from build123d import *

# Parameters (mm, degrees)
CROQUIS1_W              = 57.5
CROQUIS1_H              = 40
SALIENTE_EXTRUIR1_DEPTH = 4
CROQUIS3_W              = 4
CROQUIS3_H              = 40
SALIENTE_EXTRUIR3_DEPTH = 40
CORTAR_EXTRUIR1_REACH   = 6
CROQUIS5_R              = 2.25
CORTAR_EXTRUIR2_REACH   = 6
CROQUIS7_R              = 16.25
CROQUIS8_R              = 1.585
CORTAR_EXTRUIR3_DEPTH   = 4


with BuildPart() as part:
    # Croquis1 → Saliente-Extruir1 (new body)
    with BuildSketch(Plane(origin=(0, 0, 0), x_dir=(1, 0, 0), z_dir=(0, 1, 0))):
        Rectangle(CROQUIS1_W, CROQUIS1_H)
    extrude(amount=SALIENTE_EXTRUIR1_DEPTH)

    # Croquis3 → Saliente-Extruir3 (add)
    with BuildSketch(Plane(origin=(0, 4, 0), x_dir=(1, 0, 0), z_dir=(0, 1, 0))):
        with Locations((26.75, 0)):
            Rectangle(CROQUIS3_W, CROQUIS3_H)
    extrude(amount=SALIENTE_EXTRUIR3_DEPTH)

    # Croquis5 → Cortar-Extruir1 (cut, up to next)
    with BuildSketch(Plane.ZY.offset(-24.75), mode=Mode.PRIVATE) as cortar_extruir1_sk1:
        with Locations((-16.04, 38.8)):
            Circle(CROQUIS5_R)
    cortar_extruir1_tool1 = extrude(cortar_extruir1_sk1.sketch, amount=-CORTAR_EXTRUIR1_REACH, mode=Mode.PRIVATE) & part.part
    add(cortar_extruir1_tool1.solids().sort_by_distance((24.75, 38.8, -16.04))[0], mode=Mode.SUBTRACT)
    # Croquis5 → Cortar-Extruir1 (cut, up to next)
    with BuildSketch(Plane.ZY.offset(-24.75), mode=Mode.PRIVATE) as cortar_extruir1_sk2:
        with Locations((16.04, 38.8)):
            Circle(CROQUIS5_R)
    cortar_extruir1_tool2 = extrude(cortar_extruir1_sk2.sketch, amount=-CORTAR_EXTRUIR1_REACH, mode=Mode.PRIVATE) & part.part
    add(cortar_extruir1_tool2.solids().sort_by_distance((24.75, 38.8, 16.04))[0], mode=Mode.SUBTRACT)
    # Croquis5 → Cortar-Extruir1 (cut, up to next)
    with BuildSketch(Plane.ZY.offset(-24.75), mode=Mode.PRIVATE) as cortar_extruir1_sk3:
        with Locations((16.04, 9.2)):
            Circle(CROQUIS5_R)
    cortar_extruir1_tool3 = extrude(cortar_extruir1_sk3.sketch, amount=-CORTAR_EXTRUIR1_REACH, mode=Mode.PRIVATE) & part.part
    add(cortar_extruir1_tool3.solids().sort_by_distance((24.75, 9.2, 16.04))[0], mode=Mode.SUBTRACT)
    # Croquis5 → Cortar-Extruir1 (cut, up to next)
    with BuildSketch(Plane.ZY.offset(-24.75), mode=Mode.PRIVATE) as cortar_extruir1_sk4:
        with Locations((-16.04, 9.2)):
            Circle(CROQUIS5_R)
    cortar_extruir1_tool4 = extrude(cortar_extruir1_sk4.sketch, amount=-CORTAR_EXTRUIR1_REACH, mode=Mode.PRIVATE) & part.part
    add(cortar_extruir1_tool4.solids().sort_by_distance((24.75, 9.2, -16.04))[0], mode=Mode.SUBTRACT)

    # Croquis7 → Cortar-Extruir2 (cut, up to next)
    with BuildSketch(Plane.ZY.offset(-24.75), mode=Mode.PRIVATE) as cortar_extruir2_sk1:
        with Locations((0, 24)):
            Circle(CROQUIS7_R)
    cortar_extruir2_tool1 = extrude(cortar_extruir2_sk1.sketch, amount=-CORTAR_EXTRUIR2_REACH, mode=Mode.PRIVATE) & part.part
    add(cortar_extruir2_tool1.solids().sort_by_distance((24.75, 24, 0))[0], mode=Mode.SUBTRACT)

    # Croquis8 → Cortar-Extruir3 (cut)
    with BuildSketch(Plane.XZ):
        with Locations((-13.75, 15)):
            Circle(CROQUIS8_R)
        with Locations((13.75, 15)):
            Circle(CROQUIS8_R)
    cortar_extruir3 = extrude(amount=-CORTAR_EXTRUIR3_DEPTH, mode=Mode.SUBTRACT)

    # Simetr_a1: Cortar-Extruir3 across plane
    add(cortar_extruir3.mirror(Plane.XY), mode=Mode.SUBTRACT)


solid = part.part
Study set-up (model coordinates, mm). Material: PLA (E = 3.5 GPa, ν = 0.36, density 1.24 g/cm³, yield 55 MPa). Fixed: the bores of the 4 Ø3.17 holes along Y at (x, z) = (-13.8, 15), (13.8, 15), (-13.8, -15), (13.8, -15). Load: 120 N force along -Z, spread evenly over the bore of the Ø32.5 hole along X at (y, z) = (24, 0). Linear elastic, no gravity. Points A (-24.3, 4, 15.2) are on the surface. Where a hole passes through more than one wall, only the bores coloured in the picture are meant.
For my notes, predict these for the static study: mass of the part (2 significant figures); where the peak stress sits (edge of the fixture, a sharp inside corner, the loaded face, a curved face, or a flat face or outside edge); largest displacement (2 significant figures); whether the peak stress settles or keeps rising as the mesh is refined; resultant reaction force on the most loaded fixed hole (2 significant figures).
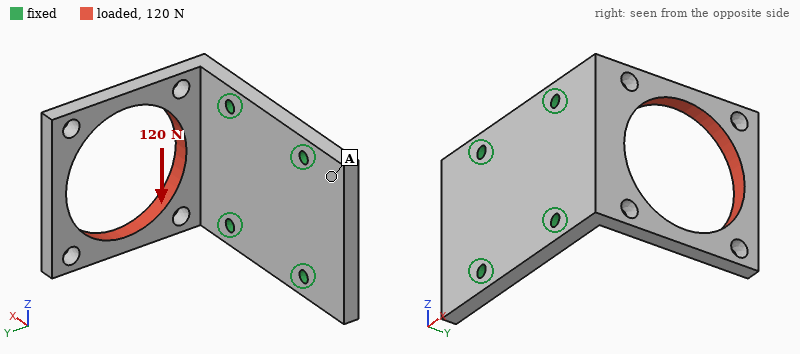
15 g
edge of the fixture
0.86 mm
keeps rising
110 N
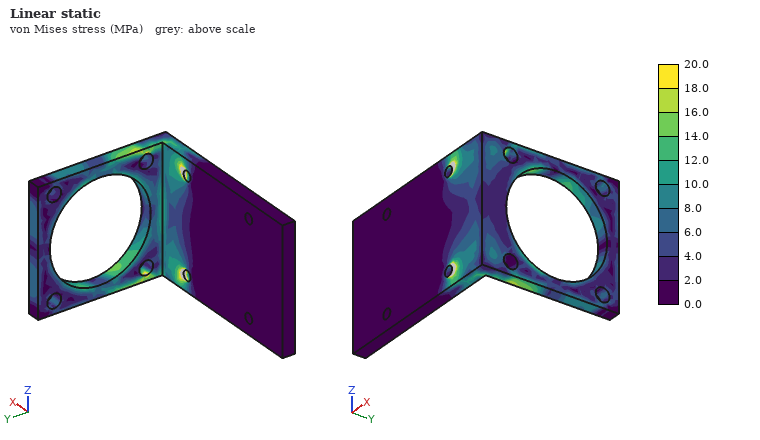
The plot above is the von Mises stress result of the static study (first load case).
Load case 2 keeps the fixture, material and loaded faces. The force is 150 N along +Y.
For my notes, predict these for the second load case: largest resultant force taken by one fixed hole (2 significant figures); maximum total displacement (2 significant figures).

84 N
0.85 mm
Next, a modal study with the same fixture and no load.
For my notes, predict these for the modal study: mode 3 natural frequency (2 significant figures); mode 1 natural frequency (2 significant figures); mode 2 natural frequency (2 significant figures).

1200 Hz
400 Hz
930 Hz
